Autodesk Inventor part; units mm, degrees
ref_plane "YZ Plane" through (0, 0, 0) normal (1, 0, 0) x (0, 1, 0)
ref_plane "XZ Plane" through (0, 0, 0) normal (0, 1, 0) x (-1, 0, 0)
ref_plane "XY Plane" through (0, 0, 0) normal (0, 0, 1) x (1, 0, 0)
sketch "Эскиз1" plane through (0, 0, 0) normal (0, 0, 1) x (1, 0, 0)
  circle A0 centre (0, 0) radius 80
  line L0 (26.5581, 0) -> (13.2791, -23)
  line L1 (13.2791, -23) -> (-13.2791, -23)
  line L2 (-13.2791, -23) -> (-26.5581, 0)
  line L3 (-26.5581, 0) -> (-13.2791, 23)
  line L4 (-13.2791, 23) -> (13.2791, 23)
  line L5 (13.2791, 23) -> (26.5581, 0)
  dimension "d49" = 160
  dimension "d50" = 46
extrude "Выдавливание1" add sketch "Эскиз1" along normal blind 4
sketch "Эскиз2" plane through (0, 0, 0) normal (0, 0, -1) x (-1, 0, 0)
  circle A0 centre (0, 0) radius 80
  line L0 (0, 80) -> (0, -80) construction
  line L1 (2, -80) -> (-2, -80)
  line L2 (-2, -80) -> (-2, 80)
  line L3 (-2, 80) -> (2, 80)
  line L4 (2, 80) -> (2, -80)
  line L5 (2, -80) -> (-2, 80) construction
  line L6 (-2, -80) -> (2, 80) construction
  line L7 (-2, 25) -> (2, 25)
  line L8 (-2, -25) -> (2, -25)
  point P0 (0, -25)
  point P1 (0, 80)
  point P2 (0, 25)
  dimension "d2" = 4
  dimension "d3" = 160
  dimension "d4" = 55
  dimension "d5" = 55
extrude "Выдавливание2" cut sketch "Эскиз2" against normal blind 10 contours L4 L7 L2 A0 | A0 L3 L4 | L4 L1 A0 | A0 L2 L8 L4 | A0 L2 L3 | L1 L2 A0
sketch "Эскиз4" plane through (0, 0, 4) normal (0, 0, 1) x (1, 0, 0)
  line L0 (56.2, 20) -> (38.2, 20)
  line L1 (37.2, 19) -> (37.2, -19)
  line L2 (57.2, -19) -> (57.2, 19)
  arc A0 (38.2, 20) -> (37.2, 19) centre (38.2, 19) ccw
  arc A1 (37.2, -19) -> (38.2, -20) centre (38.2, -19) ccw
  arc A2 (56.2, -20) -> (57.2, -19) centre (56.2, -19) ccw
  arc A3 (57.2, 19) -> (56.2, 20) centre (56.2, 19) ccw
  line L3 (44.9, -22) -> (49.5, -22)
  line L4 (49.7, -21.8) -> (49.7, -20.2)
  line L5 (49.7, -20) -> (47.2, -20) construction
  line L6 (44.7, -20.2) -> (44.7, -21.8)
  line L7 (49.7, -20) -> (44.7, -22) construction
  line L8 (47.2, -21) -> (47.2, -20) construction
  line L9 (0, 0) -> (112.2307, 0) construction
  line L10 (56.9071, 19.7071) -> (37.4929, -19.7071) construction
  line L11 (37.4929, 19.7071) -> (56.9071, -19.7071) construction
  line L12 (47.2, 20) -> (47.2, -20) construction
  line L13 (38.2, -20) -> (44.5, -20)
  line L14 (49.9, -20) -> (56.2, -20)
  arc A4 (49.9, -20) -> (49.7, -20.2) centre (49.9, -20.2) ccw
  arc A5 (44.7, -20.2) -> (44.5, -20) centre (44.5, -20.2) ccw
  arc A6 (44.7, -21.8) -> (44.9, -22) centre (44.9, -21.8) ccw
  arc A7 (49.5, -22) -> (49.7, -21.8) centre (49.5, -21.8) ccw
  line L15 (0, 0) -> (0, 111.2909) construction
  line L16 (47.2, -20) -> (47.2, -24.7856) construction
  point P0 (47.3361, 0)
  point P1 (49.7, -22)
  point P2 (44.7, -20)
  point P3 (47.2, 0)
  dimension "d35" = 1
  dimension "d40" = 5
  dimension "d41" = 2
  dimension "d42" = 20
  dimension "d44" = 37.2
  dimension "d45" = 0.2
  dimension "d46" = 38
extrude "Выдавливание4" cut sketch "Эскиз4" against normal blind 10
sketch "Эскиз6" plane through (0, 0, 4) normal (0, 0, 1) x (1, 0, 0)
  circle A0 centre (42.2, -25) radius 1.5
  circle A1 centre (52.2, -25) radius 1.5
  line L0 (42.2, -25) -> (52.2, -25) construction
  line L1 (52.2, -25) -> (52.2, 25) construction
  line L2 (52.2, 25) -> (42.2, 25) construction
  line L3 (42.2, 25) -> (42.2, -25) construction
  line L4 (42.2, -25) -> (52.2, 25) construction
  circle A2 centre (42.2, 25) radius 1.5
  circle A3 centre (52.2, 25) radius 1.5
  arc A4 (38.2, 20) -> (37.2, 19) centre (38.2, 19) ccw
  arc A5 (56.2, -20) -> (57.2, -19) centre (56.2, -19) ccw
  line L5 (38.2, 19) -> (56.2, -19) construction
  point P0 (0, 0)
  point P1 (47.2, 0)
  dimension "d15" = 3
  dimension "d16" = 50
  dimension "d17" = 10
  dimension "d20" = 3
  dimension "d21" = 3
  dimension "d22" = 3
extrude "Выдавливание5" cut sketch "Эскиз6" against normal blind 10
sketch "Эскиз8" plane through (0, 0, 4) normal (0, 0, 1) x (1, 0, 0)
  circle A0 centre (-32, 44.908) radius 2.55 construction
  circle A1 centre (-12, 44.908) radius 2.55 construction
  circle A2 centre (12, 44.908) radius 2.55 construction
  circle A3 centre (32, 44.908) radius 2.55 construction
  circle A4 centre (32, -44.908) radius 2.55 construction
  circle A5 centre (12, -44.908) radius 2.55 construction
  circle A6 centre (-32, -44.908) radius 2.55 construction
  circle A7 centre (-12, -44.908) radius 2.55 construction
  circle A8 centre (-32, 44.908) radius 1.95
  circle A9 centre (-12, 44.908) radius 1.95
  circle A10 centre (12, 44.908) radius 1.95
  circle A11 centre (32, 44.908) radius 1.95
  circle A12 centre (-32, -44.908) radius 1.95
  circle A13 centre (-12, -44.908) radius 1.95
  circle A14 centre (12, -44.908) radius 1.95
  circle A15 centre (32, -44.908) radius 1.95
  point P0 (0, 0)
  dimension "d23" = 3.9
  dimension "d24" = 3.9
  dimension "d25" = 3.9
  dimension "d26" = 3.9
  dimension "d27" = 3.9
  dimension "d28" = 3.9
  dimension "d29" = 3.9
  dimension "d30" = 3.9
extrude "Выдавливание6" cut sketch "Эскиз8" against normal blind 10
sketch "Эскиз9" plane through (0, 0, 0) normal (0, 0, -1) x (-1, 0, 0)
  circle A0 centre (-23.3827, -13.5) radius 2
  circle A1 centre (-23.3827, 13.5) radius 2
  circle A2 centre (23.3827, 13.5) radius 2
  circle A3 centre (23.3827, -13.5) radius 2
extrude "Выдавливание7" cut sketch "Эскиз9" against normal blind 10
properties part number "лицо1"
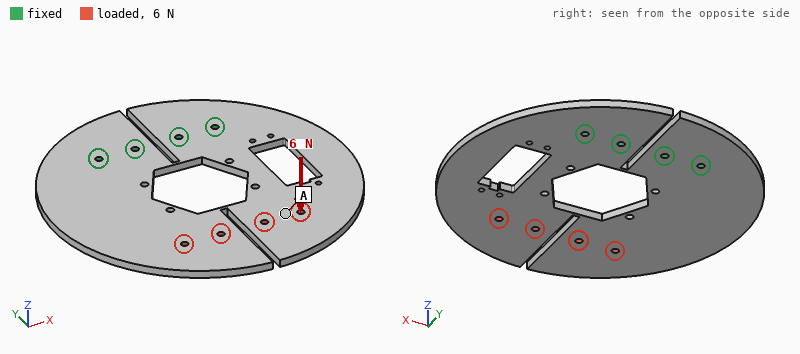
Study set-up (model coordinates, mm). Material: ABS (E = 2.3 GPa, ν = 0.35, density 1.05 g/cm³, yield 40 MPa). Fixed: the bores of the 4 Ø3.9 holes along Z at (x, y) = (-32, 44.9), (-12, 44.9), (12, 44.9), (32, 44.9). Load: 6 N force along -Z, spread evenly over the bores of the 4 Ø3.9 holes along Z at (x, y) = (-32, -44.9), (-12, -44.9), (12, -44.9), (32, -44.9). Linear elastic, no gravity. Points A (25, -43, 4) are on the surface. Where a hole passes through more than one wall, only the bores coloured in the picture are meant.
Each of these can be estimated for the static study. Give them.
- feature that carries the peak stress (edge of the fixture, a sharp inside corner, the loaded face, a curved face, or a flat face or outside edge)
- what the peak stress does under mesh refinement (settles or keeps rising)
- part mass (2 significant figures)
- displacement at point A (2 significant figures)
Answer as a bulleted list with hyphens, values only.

- edge of the fixture
- keeps rising
- 71 g
- 1.3 mm
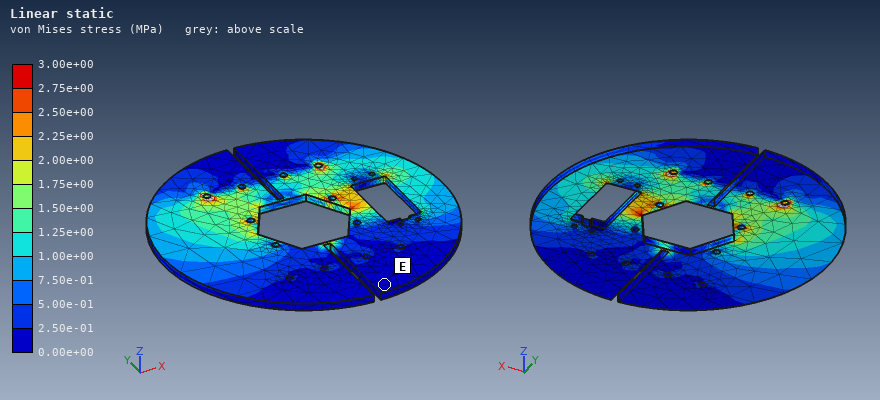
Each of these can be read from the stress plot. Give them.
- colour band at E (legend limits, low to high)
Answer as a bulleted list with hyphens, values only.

- 0.00e+00 to 2.50e-01 MPa
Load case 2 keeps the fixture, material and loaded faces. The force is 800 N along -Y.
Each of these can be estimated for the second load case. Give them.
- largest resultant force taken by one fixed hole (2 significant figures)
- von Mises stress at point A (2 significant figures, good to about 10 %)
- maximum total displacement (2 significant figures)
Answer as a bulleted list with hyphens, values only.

- 350 N
- 2.1 MPa
- 0.51 mm
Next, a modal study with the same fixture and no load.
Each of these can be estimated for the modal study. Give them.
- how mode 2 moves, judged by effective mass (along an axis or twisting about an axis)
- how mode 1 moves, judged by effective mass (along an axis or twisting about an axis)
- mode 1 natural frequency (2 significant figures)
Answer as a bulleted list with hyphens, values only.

- twisting about Y
- along Z
- 60 Hz
